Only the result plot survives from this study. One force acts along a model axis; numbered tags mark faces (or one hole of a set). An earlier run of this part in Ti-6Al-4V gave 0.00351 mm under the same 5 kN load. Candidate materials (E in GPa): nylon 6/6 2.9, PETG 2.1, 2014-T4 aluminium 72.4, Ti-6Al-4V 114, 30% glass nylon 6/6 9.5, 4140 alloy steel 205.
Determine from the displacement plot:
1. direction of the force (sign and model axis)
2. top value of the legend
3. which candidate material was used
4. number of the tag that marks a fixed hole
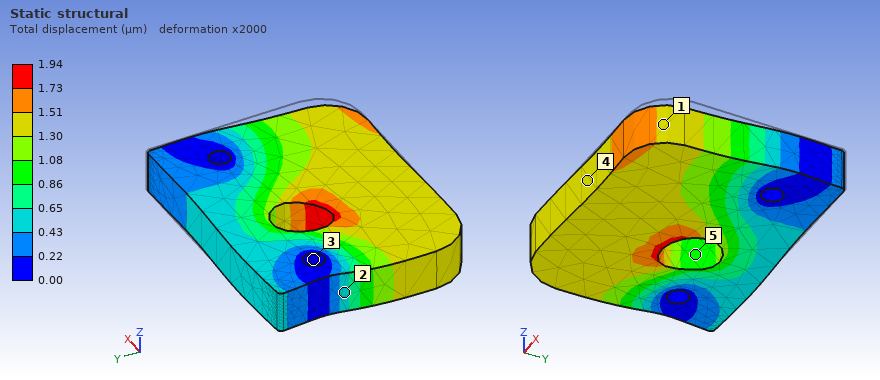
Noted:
-X
1.94 µm
4140 alloy steel
3
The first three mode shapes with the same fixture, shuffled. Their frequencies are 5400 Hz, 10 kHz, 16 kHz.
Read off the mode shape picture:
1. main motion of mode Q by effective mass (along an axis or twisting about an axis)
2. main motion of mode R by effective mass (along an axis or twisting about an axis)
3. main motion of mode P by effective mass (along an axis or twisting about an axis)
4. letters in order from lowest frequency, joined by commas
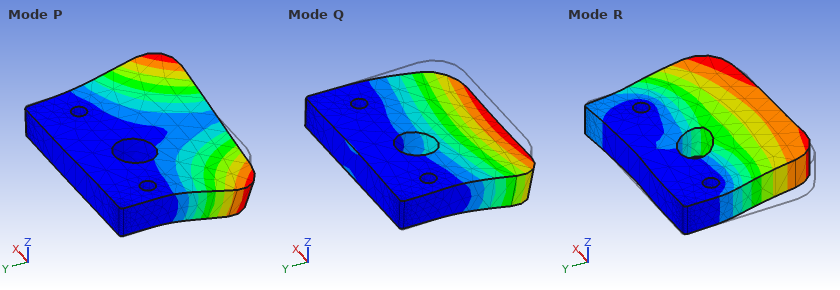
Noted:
along Z
along X
twisting about Y
Q, P, R
